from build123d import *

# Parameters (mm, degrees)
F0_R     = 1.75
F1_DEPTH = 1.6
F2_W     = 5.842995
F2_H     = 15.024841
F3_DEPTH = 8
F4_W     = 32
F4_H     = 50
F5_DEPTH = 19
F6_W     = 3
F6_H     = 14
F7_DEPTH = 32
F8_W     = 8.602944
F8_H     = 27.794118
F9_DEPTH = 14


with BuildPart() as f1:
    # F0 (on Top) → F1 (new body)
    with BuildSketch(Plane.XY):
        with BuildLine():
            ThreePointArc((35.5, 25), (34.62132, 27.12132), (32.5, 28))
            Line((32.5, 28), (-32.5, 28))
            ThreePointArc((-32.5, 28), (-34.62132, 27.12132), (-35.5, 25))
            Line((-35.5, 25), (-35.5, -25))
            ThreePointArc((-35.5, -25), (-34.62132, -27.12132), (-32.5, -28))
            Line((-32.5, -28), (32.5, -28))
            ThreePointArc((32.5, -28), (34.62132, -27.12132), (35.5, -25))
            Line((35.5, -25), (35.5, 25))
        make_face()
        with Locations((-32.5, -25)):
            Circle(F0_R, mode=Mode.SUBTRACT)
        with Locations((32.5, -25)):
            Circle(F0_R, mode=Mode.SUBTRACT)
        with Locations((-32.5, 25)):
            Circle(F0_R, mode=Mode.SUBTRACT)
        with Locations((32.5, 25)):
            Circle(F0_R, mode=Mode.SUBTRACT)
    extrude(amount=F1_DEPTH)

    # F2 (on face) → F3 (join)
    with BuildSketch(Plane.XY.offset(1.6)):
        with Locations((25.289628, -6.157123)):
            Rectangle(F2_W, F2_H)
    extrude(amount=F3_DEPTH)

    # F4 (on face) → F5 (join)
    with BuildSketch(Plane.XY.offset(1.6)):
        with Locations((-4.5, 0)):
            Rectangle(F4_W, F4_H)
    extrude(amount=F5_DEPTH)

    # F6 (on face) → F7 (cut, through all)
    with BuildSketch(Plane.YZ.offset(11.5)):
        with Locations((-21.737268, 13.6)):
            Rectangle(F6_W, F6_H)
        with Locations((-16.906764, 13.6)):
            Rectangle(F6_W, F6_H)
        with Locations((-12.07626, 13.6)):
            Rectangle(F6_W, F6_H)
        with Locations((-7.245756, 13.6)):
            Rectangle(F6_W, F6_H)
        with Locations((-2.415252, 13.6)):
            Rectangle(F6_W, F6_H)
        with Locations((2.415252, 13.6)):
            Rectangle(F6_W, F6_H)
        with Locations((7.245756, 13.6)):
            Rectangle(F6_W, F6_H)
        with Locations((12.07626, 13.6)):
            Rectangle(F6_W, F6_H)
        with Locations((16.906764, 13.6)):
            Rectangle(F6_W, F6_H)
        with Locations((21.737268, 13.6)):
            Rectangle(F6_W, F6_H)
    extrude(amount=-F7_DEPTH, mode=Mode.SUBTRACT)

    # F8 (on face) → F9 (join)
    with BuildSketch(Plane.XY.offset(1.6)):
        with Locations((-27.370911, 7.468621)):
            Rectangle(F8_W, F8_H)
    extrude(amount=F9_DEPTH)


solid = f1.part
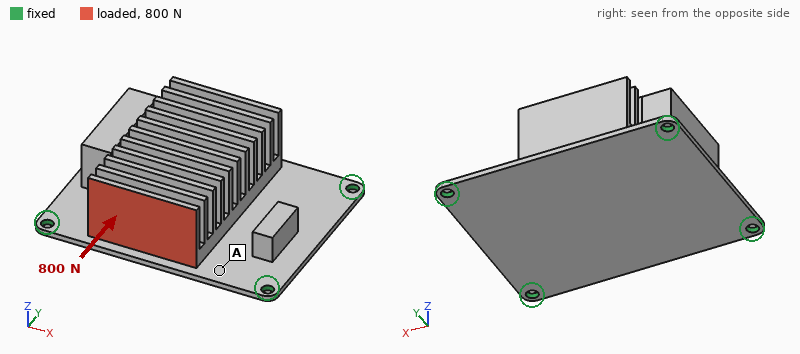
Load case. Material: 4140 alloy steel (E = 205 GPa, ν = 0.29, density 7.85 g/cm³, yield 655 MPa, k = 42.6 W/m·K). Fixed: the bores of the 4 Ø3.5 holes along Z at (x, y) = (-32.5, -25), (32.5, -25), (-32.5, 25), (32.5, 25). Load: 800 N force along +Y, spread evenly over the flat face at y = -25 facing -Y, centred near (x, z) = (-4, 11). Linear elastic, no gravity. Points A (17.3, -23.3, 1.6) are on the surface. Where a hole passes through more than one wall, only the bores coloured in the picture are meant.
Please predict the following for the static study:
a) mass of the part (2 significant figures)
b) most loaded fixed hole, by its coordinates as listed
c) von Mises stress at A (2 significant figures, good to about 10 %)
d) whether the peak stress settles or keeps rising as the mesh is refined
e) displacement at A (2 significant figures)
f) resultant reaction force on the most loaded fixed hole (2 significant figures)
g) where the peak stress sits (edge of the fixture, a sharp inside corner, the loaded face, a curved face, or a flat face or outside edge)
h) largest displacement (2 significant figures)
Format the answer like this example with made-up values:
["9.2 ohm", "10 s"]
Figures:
["210 g", "(-32.5, 25)", "23 MPa", "keeps rising", "0.017 mm", "440 N", "edge of the fixture", "0.10 mm"]
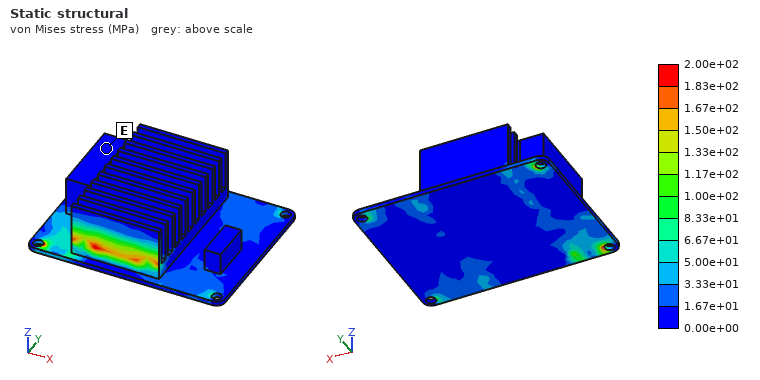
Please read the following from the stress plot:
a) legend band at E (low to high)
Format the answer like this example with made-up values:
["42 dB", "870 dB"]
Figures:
["0.00e+00 to 1.67e+01 MPa"]
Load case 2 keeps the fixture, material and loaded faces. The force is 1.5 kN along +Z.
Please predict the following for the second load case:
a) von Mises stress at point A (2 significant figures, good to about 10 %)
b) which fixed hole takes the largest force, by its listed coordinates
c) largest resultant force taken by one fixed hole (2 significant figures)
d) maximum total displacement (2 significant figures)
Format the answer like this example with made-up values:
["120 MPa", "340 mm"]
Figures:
["290 MPa", "(-32.5, -25)", "1.2 kN", "0.33 mm"]
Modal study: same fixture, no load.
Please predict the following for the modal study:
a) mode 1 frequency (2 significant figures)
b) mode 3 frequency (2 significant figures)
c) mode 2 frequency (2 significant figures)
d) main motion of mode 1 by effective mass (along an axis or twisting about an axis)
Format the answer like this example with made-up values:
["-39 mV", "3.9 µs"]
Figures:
["1200 Hz", "2800 Hz", "2000 Hz", "along Z"]
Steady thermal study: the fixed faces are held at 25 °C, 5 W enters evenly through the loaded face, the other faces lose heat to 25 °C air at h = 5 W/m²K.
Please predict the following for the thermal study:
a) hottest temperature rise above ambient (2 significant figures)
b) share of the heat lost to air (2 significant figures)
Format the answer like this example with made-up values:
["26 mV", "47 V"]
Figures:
["33 K", "25 %"]
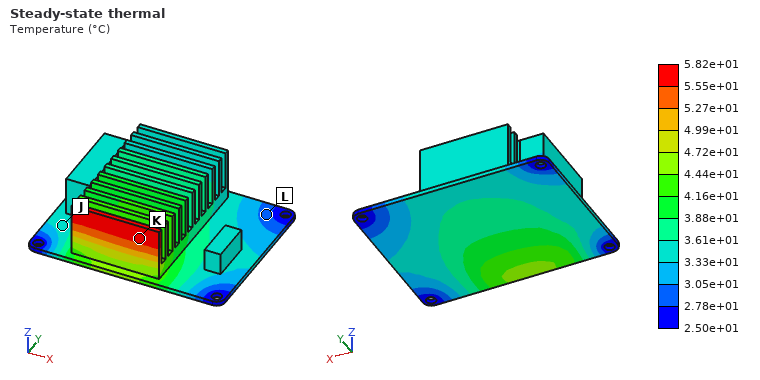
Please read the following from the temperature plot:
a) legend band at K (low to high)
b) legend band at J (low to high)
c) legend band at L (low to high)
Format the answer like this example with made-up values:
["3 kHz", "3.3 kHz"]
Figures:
["5.55e+01 to 5.82e+01 °C", "3.33e+01 to 3.61e+01 °C", "2.78e+01 to 3.05e+01 °C"]
